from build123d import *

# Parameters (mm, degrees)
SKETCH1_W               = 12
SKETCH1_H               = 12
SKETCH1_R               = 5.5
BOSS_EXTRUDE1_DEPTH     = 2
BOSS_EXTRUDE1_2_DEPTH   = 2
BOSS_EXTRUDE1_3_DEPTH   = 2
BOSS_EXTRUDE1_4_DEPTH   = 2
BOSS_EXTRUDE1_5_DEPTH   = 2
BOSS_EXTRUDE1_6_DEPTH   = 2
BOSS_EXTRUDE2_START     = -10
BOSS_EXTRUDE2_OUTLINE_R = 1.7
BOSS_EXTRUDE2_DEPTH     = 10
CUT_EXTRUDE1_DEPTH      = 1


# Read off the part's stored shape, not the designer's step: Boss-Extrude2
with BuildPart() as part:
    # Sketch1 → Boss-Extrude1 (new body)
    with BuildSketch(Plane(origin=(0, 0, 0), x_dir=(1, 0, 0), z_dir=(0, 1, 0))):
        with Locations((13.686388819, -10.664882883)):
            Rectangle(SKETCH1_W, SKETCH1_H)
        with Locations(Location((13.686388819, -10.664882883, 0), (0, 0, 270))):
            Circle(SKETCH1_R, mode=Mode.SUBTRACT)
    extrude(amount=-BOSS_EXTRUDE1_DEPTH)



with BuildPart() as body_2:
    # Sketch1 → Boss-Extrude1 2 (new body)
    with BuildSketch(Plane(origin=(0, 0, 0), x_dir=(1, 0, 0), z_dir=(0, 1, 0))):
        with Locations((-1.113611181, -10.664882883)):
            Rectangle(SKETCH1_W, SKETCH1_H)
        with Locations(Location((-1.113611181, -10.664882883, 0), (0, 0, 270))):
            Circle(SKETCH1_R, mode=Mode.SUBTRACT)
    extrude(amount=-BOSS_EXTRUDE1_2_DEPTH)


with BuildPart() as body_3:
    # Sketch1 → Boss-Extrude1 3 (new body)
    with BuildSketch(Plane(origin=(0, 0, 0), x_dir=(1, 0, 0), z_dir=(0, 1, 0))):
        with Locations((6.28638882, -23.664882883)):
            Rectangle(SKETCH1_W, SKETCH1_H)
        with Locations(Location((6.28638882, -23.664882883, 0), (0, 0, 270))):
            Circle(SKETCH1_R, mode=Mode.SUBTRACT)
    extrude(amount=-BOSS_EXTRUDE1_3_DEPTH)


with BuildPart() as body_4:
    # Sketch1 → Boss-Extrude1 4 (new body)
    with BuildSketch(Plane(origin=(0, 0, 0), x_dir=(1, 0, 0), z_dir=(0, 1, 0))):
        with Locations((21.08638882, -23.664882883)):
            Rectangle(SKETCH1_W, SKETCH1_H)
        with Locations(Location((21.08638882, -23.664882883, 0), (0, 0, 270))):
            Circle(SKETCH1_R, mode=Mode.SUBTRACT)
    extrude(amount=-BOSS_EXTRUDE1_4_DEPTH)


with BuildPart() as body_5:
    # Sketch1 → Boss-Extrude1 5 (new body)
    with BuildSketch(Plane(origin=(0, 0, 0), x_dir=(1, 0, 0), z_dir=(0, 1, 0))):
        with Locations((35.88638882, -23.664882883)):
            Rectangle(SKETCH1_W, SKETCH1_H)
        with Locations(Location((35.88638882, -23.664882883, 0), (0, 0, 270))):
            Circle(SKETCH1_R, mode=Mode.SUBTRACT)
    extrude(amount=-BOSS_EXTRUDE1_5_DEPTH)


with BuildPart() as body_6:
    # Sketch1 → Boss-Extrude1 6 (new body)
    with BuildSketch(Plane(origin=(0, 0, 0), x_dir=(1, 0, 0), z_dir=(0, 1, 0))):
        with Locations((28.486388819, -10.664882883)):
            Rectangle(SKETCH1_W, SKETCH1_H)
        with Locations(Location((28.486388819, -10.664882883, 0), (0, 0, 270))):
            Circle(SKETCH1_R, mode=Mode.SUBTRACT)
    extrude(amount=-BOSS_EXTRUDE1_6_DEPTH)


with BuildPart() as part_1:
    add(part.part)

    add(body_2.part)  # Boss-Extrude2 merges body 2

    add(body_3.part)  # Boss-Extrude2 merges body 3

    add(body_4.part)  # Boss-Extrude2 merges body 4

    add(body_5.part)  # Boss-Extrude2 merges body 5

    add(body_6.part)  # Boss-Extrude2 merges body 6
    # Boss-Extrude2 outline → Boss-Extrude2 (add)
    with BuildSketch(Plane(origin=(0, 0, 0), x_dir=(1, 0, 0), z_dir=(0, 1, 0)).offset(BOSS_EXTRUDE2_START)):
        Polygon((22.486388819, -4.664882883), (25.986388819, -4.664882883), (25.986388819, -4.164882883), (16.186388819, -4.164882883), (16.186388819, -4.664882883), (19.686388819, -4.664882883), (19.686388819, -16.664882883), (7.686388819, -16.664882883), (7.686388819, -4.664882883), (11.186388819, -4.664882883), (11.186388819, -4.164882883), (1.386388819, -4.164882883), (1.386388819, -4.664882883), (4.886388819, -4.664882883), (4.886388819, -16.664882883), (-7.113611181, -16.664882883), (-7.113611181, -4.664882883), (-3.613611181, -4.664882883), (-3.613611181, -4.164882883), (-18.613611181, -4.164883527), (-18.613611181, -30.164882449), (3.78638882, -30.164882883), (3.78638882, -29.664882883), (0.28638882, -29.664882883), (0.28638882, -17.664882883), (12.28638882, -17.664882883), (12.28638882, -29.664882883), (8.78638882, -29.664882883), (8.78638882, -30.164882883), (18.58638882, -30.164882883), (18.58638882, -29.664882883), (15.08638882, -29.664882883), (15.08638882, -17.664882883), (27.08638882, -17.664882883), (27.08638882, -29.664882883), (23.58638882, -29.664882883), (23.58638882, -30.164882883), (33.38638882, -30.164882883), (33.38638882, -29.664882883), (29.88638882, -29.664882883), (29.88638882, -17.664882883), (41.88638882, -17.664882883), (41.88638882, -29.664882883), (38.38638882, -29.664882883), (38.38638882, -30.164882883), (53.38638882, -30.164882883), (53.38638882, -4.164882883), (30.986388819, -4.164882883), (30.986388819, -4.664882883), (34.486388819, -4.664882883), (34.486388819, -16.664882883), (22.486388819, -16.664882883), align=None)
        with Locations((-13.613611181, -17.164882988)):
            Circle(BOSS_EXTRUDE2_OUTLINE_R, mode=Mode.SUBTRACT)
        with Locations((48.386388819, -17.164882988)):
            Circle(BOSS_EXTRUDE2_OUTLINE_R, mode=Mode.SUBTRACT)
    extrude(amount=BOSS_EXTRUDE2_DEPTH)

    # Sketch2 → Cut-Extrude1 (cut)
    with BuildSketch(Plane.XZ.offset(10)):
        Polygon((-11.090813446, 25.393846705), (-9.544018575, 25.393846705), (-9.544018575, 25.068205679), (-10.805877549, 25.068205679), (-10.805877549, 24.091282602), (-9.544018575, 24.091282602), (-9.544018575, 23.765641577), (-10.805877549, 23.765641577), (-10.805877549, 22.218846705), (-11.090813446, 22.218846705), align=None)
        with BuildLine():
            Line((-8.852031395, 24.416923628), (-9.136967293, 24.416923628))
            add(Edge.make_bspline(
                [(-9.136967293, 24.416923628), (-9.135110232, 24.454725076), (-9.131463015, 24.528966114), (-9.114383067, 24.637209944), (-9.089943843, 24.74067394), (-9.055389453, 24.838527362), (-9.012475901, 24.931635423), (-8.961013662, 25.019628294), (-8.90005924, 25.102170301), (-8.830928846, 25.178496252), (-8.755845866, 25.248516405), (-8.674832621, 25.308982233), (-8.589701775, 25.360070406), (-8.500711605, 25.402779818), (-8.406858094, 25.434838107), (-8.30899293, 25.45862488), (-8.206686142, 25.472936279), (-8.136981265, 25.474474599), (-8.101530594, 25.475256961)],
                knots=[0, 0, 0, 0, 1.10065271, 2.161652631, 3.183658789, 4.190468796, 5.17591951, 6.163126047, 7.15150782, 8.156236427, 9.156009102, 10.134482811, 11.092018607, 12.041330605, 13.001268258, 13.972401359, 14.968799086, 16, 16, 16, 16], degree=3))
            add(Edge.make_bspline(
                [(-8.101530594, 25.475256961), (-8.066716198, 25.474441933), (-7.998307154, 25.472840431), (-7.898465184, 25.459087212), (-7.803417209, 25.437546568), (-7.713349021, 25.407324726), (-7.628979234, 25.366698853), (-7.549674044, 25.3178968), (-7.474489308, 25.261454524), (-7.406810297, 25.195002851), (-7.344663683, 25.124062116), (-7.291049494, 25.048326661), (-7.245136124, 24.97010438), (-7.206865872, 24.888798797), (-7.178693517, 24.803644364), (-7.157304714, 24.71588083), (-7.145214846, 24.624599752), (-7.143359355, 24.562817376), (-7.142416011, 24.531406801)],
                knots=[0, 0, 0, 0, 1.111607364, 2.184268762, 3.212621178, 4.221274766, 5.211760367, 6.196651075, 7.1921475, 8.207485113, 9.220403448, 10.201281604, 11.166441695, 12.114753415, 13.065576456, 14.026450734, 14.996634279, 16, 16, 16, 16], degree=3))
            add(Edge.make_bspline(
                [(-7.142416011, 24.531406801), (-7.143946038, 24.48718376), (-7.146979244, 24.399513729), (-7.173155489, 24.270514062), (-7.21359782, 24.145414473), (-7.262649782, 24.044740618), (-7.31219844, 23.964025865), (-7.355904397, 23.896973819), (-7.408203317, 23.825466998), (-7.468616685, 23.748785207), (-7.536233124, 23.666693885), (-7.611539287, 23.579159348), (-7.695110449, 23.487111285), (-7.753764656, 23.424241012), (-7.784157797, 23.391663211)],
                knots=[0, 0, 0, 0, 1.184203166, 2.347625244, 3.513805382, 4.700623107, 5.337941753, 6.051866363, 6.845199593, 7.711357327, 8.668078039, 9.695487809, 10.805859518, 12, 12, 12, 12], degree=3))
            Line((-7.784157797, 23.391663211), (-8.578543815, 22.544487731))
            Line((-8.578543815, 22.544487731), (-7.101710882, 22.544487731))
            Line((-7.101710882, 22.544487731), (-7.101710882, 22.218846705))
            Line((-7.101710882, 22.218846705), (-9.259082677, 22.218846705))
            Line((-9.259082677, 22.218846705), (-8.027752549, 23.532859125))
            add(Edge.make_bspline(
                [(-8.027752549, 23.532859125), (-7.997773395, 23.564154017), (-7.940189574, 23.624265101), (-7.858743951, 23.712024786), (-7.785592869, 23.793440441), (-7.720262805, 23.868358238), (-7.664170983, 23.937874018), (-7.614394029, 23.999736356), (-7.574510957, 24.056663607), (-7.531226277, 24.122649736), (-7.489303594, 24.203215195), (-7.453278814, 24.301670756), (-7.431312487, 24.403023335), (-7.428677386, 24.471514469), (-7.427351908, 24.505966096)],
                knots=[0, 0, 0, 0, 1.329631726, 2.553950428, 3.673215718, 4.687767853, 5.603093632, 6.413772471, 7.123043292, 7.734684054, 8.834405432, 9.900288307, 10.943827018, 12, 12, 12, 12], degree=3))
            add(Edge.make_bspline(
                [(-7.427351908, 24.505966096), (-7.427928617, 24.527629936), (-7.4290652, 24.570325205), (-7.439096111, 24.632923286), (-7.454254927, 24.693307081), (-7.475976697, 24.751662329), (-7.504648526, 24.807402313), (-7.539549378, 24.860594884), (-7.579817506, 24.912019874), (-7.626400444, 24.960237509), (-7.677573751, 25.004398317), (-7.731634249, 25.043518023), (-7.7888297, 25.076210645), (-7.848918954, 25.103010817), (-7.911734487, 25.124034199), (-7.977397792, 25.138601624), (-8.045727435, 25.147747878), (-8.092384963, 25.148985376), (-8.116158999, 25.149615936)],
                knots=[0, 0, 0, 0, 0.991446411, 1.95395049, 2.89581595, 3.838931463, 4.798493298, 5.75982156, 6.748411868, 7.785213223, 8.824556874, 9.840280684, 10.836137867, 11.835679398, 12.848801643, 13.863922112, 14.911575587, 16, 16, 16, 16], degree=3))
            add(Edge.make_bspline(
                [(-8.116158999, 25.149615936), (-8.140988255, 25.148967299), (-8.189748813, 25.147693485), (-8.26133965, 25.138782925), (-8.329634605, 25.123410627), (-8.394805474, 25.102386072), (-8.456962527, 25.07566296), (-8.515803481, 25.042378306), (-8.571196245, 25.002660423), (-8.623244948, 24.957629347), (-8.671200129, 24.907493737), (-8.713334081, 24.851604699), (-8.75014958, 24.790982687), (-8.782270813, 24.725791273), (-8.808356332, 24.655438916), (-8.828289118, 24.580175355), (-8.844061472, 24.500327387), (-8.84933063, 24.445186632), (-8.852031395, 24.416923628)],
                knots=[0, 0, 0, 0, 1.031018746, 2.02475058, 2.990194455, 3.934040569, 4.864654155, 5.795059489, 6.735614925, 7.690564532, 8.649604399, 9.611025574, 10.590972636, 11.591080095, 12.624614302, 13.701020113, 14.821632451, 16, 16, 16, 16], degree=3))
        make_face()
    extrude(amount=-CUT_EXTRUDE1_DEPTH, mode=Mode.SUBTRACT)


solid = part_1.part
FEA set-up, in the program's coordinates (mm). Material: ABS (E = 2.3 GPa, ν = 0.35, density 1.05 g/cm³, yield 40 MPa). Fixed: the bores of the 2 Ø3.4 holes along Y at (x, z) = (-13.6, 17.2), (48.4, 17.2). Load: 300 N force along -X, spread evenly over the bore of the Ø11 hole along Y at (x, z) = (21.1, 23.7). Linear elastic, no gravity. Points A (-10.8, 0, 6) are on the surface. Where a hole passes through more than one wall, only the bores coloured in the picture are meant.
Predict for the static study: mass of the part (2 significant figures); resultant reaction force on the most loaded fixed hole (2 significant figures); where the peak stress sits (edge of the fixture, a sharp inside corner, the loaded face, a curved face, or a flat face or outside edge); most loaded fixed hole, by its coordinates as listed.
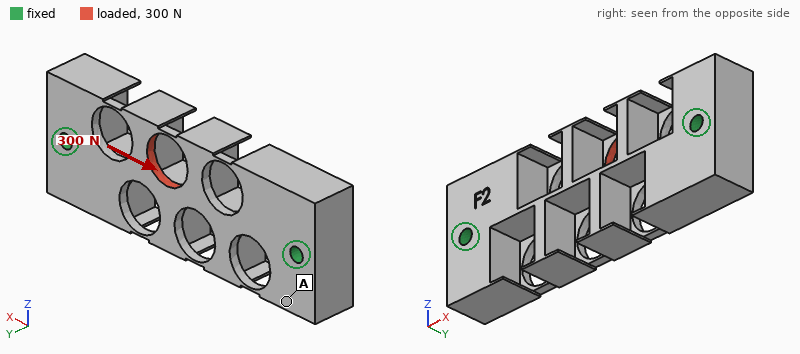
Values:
11 g
180 N
a curved face
(48.4, 17.2)
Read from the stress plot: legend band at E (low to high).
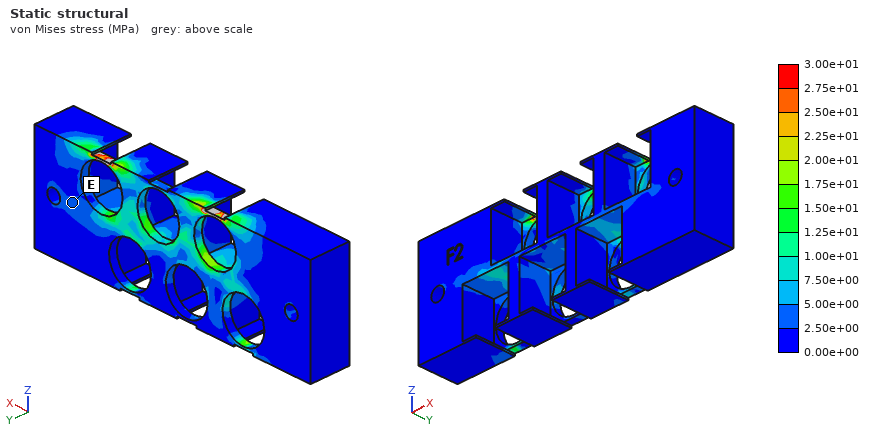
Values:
2.50e+00 to 5.00e+00 MPa
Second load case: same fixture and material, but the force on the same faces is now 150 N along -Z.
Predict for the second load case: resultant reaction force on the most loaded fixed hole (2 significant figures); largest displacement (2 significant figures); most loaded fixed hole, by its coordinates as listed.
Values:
90 N
0.40 mm
(48.4, 17.2)
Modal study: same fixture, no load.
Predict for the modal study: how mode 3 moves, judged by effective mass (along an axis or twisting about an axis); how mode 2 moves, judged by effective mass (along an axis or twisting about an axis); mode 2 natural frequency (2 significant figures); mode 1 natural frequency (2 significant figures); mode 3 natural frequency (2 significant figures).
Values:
along Z
along Y
2300 Hz
1800 Hz
2500 Hz
